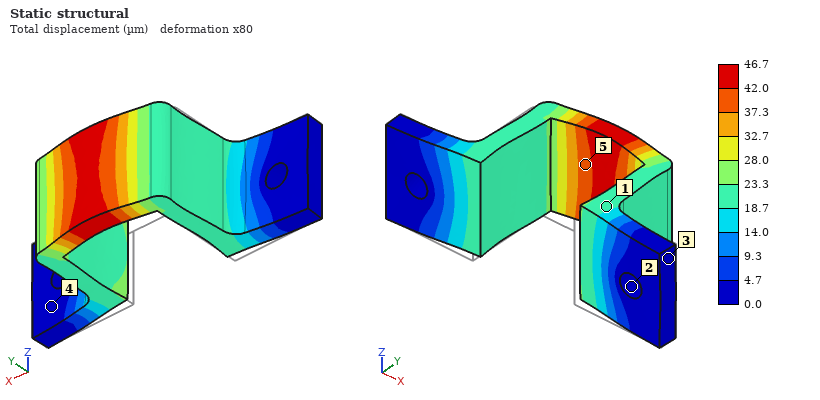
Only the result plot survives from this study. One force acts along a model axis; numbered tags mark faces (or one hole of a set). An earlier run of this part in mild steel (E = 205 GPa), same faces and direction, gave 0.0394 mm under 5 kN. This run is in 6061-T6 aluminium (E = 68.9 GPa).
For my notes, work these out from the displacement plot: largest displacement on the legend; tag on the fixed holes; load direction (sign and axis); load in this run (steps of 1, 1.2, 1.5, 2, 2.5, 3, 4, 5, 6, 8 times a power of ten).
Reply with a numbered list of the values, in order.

1. 46.7 µm
2. 2
3. +Y
4. 2 kN
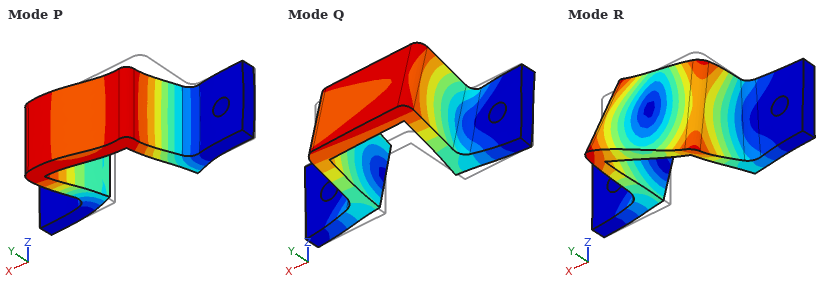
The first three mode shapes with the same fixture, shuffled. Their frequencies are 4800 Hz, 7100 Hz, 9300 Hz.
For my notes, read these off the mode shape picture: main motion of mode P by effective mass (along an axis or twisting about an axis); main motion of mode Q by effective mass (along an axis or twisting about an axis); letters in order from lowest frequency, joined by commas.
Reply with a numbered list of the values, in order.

1. along X
2. along Z
3. Q, P, R
